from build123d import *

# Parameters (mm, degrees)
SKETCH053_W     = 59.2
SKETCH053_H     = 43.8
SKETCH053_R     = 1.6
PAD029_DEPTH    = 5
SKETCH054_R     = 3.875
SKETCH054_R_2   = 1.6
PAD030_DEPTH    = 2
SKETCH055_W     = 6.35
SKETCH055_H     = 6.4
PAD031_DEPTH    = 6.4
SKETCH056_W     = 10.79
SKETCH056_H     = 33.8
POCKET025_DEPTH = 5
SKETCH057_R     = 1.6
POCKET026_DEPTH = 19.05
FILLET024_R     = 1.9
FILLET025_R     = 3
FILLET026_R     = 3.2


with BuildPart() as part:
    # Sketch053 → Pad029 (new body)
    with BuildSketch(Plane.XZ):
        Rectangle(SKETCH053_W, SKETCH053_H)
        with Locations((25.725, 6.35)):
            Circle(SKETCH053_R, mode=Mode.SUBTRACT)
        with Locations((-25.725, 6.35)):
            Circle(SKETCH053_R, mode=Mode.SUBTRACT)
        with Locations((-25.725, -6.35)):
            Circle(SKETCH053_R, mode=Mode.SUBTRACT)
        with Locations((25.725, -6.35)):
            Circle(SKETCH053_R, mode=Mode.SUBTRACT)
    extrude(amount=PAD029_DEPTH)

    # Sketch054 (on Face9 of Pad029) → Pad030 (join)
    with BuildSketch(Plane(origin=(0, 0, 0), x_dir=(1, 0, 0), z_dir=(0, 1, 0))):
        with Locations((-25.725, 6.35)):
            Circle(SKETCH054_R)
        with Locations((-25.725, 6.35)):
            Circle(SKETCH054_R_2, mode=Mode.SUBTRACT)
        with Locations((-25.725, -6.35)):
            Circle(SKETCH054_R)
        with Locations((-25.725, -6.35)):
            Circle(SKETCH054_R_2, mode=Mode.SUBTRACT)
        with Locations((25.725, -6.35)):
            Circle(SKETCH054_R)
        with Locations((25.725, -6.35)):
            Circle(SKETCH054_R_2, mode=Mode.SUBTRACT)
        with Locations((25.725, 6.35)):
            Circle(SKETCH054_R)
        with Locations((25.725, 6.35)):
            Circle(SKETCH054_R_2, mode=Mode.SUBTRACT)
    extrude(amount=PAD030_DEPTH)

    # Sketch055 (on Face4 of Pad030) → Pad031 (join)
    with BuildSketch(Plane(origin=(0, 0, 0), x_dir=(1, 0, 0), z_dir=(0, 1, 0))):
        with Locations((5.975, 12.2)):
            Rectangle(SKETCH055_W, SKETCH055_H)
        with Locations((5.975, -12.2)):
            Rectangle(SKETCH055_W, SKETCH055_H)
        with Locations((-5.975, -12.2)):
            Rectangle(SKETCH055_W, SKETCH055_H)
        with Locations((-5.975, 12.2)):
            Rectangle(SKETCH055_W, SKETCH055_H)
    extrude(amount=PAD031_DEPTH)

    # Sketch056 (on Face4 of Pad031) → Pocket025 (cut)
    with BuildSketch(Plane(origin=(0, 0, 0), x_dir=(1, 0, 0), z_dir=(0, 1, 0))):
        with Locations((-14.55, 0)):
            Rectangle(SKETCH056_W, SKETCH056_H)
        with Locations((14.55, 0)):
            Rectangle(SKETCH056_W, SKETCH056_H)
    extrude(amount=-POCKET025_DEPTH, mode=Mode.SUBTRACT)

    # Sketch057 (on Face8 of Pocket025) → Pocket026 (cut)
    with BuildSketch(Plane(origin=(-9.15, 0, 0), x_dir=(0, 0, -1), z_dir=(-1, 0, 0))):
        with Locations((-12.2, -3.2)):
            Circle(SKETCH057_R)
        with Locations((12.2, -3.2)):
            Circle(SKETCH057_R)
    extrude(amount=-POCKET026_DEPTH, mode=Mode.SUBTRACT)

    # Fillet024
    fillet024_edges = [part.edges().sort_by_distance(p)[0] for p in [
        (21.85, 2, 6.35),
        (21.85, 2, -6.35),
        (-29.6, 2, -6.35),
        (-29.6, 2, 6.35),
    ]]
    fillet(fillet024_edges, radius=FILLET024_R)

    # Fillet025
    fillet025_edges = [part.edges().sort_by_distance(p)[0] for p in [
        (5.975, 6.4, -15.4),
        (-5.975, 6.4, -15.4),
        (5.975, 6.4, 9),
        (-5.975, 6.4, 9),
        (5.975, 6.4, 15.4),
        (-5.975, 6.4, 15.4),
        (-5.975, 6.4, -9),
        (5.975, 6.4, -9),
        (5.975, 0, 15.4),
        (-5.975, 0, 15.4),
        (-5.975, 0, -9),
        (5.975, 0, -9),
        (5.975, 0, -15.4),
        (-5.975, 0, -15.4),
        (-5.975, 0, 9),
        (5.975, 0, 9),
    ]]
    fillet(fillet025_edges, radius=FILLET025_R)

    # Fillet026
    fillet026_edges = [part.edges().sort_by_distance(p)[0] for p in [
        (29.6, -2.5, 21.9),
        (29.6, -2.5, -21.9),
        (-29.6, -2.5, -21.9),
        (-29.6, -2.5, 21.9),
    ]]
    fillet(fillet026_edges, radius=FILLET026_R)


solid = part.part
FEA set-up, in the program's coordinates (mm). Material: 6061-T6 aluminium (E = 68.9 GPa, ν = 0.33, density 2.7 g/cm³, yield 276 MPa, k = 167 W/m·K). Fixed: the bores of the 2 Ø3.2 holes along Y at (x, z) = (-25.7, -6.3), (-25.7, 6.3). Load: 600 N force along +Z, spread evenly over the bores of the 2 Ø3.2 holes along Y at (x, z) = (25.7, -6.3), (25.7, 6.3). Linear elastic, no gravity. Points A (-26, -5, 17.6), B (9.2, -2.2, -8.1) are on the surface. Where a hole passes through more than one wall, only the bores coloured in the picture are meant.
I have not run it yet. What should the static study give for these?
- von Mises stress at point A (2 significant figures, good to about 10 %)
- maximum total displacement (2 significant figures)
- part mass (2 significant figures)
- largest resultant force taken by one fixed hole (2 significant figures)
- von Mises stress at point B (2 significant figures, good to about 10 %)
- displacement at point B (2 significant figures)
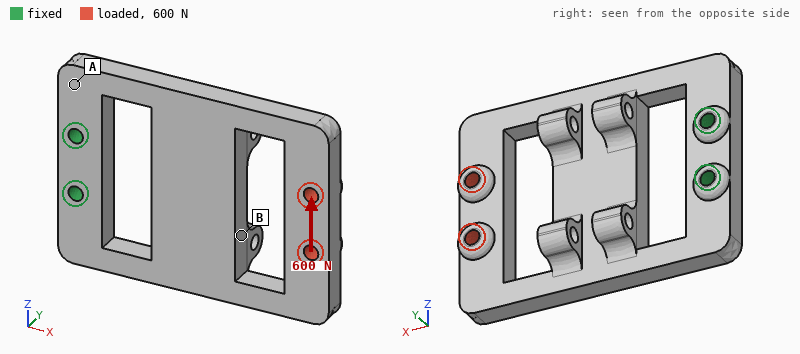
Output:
46 MPa
0.26 mm
28 g
1.4 kN
17 MPa
0.15 mm
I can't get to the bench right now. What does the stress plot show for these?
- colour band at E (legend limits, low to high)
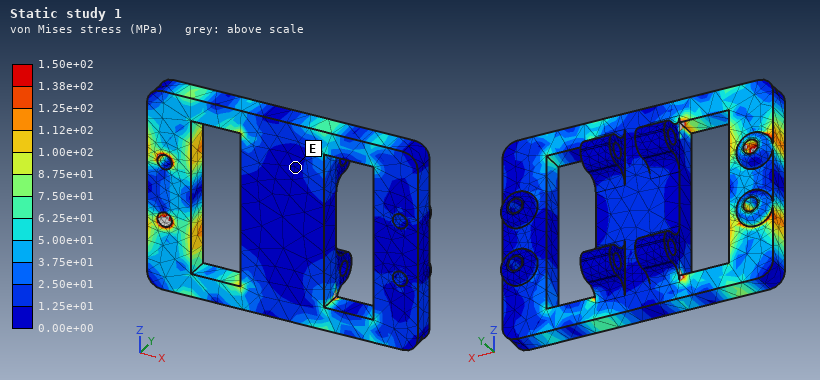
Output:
0.00e+00 to 1.25e+01 MPa
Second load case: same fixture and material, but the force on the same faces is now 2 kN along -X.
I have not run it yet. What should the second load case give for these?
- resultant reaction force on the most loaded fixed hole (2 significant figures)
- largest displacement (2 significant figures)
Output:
1.2 kN
0.42 mm
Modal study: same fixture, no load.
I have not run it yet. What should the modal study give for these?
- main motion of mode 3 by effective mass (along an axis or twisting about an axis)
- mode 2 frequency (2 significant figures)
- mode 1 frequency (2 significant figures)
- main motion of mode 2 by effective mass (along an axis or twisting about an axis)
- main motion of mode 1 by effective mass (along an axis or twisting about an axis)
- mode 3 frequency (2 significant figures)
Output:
twisting about X
2400 Hz
690 Hz
along Z
along Y
2600 Hz
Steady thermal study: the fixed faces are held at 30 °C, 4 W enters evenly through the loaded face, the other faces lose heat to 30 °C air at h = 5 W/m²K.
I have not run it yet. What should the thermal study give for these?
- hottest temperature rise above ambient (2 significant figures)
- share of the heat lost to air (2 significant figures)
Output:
22 K
8.5 %
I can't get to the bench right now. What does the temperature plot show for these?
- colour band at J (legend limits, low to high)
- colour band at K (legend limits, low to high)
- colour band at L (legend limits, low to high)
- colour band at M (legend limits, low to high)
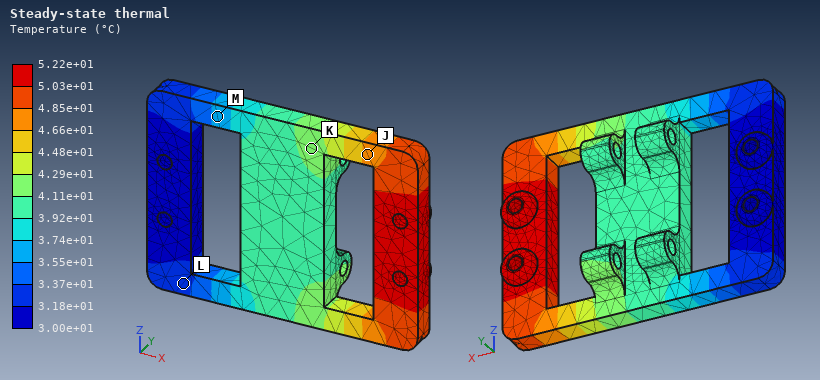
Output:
4.66e+01 to 4.85e+01 °C
4.11e+01 to 4.29e+01 °C
3.18e+01 to 3.37e+01 °C
3.55e+01 to 3.74e+01 °C
